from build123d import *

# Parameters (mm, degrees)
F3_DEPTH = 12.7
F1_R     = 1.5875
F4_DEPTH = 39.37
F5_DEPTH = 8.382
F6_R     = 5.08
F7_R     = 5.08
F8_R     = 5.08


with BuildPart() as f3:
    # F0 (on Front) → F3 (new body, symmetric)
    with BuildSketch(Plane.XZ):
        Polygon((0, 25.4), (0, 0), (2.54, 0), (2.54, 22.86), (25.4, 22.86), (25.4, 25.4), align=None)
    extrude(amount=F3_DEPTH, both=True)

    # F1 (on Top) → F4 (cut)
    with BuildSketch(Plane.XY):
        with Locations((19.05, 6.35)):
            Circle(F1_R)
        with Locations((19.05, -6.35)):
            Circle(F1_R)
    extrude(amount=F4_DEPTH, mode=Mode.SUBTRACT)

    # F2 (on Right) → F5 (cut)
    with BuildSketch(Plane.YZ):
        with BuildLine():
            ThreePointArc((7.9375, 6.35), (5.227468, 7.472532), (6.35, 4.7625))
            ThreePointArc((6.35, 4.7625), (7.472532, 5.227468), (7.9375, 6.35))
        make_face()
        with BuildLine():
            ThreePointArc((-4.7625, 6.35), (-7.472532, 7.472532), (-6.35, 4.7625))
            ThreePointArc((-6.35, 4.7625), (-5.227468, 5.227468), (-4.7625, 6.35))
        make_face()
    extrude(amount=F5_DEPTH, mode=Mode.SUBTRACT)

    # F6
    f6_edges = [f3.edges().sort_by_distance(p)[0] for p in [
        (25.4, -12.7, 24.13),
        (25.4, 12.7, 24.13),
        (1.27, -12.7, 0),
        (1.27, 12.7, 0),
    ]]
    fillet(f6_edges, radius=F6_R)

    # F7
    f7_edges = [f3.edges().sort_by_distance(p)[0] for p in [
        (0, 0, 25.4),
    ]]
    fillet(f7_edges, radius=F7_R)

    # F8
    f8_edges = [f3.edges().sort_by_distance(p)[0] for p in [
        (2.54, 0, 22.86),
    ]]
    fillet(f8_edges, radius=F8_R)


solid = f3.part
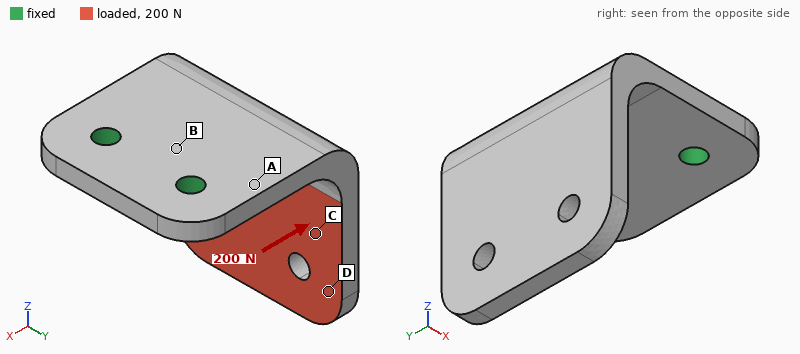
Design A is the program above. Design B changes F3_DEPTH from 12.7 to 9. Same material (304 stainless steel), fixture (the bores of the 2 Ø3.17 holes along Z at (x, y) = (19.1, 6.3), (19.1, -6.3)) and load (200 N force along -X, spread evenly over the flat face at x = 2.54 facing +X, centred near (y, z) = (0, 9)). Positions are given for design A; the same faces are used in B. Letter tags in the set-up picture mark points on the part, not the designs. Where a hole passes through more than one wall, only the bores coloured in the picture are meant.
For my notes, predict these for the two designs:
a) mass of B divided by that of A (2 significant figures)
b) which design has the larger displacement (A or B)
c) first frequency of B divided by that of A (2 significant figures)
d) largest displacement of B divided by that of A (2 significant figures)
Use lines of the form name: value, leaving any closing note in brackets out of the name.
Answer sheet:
mass of B divided by that of A: 0.70
which design has the larger displacement: B
first frequency of B divided by that of A: 1.0
largest displacement of B divided by that of A: 1.4
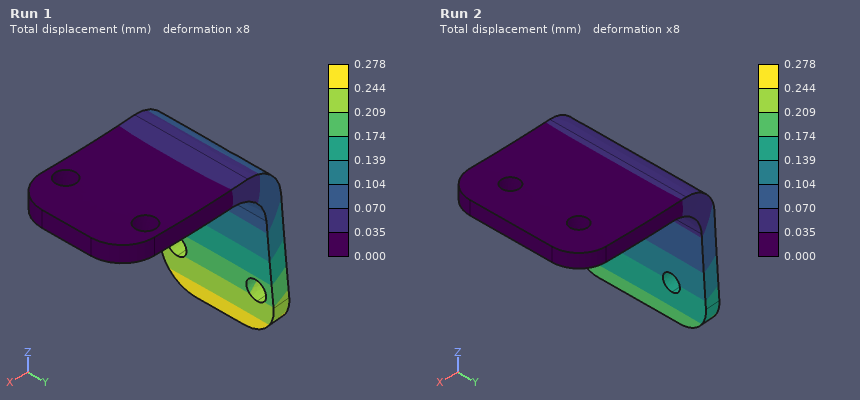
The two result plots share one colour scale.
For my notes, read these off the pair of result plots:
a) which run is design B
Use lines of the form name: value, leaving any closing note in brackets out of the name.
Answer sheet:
which run is design B: Run 1
